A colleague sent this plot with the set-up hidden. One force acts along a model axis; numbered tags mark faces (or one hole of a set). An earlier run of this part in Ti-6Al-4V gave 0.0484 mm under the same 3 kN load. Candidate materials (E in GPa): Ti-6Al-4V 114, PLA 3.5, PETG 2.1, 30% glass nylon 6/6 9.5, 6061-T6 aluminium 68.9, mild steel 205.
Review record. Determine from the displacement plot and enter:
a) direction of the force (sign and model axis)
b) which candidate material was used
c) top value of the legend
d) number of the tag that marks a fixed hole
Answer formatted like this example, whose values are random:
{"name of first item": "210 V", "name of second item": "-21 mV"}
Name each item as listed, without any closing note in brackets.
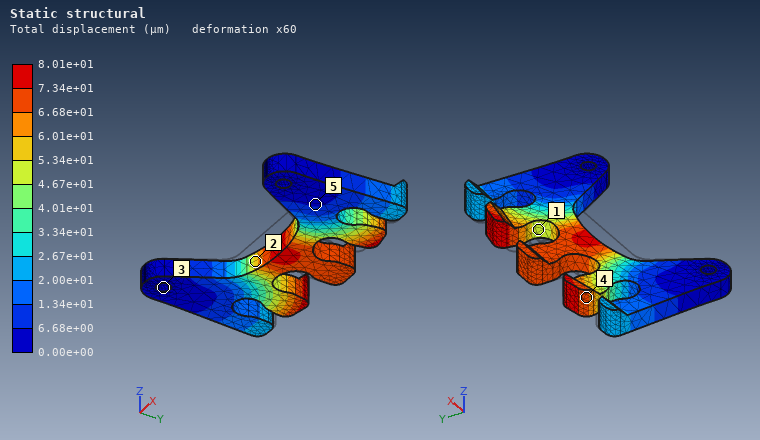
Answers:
{"direction of the force": "+Y", "which candidate material was used": "6061-T6 aluminium", "top value of the legend": "8.01e+01 µm", "number of the tag that marks a fixed hole": "3"}
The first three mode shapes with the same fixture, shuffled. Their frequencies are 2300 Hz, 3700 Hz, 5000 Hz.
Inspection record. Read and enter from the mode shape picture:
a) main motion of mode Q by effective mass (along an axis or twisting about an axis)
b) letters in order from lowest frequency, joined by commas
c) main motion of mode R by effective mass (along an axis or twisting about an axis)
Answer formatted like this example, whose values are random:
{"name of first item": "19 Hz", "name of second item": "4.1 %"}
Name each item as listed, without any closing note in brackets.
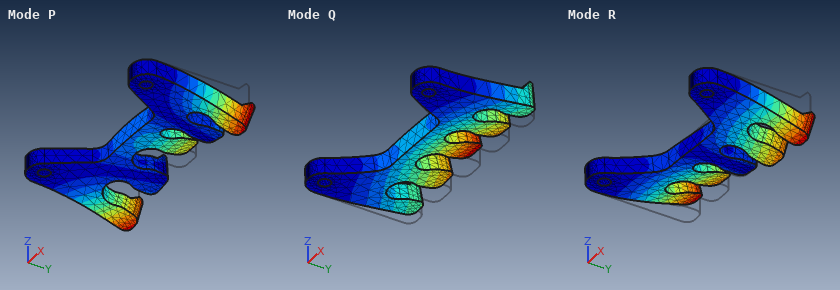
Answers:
{"main motion of mode Q by effective mass": "along Z", "letters in order from lowest frequency, joined by commas": "Q, R, P", "main motion of mode R by effective mass": "twisting about Y"}
